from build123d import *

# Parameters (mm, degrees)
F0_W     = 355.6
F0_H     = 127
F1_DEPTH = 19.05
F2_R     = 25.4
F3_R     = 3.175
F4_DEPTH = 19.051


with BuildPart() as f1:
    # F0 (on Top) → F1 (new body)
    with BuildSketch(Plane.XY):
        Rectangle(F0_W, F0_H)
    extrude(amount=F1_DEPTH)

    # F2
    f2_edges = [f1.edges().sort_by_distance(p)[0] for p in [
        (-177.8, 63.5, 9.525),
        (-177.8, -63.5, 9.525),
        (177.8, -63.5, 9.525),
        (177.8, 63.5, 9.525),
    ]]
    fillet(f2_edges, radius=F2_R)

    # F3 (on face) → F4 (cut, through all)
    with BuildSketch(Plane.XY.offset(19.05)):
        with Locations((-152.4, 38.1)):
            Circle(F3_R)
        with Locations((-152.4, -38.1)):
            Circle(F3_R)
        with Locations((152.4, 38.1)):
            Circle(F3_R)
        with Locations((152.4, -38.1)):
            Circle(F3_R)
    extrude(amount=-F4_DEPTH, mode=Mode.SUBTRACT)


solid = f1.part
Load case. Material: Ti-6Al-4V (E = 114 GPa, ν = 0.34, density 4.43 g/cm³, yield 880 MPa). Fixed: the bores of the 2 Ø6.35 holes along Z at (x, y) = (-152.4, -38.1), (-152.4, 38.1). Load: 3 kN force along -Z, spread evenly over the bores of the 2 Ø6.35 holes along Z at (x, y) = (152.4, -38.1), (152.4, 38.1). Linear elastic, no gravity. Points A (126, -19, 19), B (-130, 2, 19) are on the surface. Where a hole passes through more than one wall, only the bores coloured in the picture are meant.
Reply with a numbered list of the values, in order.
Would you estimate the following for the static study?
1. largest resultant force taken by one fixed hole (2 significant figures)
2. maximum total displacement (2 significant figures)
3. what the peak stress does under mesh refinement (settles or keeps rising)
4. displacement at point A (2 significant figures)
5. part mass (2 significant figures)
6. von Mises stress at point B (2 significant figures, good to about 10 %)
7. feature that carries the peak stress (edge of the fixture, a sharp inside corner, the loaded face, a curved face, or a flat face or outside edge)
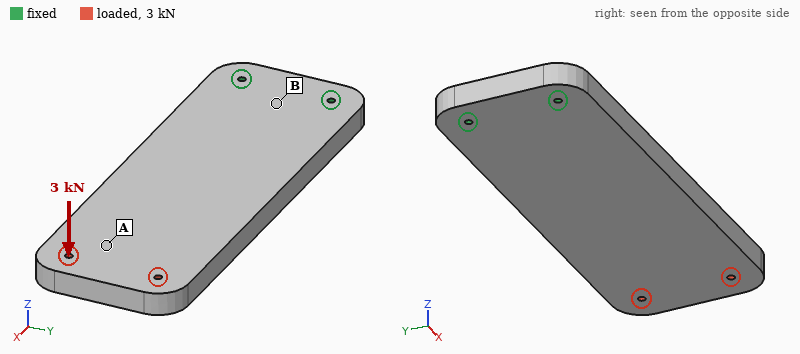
1. 1.5 kN
2. 4.2 mm
3. keeps rising
4. 3.3 mm
5. 3.8 kg
6. 90 MPa
7. edge of the fixture
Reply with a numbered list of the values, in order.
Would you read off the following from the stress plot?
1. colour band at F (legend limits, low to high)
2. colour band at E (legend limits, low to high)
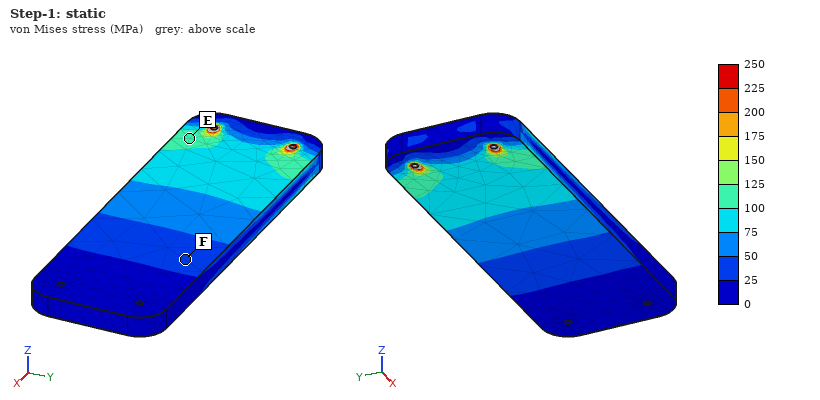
1. 25 to 50 MPa
2. 100 to 125 MPa
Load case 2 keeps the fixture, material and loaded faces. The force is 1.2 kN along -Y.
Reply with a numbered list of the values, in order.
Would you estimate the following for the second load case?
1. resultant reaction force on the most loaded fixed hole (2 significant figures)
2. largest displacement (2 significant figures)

1. 4.7 kN
2. 48 µm
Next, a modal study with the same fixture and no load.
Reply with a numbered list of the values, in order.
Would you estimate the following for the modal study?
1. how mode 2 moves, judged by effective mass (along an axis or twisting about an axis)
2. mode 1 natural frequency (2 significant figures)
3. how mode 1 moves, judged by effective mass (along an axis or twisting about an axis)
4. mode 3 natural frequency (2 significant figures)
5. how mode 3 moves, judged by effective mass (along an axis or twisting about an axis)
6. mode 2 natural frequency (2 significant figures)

1. twisting about X
2. 140 Hz
3. along Z
4. 770 Hz
5. along Y
6. 730 Hz
